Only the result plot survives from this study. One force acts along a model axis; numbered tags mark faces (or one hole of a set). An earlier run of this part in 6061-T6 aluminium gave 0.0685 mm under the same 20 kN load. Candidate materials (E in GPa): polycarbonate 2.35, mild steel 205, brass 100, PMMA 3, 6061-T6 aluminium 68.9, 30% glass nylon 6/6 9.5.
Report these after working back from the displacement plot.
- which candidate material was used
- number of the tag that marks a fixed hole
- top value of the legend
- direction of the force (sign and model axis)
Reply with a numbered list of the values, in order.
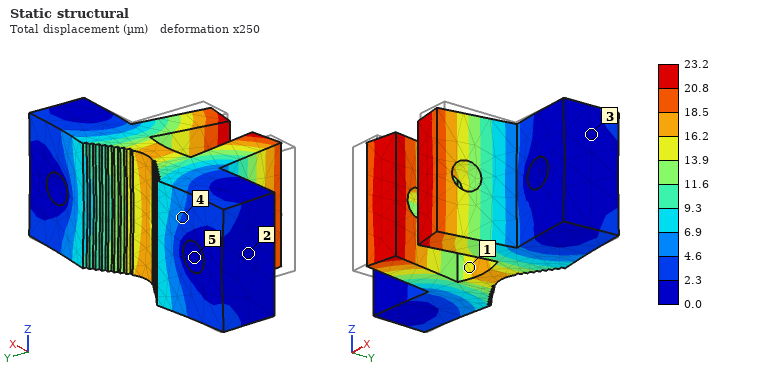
1. mild steel
2. 5
3. 23.2 µm
4. +Y
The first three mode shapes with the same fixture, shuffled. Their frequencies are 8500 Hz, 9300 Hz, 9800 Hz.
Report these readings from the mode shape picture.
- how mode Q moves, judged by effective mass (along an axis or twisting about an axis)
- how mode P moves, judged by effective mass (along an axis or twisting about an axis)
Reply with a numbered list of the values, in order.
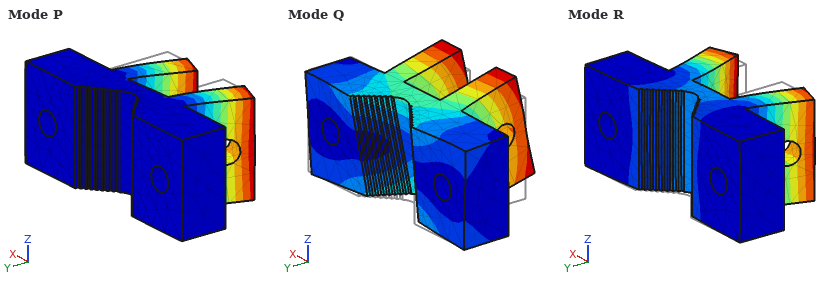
1. along Z
2. along X
